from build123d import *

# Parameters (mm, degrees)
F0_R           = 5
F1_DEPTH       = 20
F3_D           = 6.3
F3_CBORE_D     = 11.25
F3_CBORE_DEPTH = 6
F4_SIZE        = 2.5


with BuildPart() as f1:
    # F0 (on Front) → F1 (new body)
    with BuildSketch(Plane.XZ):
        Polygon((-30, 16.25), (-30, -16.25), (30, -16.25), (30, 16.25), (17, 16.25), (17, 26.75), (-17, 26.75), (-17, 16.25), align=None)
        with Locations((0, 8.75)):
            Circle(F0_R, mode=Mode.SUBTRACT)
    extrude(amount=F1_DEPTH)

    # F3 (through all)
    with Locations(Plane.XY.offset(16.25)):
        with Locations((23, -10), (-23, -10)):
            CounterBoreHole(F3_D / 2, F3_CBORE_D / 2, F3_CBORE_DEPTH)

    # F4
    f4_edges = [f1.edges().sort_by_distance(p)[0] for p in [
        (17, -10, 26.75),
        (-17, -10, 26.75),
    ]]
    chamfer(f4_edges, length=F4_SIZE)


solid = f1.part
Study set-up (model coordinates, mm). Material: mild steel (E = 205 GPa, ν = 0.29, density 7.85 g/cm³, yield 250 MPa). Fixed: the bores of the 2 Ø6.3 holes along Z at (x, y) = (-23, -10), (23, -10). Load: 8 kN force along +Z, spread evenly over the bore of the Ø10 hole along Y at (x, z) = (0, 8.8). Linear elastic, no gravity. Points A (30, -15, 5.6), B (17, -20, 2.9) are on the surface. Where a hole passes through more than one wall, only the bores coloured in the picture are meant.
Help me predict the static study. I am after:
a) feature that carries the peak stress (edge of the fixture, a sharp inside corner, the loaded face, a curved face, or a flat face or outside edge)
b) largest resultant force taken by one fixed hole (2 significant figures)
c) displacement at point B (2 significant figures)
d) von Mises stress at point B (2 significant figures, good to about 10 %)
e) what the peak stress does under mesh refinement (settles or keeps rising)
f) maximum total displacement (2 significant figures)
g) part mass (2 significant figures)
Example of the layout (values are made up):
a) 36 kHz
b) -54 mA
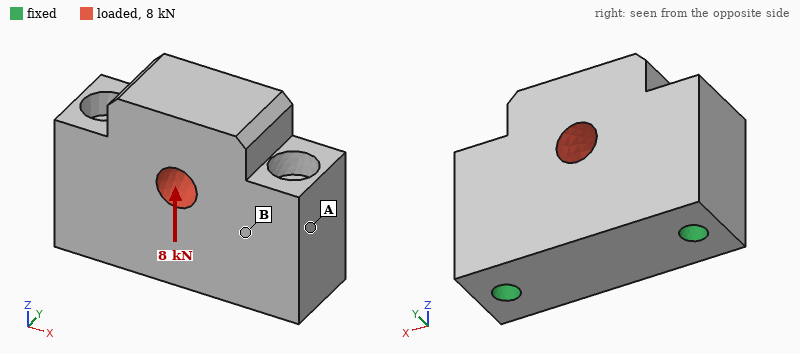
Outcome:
a) edge of the fixture
b) 4.2 kN
c) 0.71 µm
d) 10 MPa
e) keeps rising
f) 2.3 µm
g) 330 g
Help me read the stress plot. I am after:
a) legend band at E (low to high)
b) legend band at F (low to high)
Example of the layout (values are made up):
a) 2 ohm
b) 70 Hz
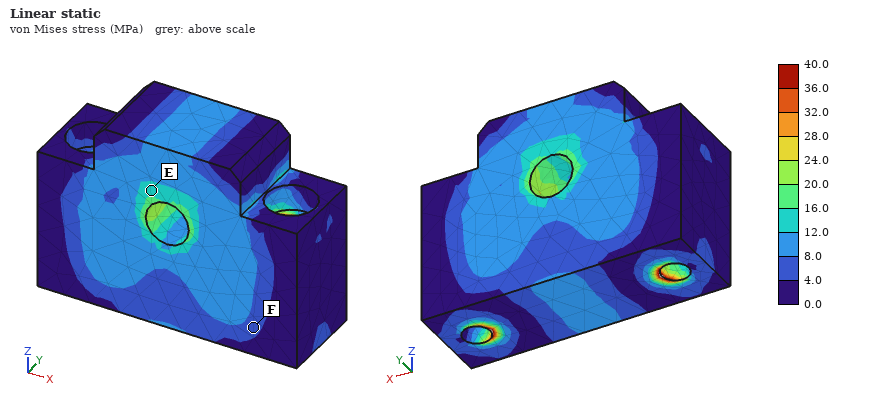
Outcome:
a) 12.0 to 16.0 MPa
b) 4.0 to 8.0 MPa
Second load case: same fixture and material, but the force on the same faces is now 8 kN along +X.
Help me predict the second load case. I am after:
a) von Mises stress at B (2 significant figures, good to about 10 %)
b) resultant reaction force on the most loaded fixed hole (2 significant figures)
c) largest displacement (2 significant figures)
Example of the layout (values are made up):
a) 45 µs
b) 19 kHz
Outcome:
a) 5.7 MPa
b) 4.2 kN
c) 1.8 µm
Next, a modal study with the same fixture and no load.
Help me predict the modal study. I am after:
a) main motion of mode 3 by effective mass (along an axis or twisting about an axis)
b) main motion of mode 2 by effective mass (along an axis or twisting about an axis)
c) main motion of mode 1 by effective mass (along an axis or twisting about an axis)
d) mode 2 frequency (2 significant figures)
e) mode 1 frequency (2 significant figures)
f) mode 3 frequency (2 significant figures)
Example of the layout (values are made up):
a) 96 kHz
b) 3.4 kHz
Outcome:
a) along Z
b) along Y
c) along Y
d) 25 kHz
e) 14 kHz
f) 27 kHz
